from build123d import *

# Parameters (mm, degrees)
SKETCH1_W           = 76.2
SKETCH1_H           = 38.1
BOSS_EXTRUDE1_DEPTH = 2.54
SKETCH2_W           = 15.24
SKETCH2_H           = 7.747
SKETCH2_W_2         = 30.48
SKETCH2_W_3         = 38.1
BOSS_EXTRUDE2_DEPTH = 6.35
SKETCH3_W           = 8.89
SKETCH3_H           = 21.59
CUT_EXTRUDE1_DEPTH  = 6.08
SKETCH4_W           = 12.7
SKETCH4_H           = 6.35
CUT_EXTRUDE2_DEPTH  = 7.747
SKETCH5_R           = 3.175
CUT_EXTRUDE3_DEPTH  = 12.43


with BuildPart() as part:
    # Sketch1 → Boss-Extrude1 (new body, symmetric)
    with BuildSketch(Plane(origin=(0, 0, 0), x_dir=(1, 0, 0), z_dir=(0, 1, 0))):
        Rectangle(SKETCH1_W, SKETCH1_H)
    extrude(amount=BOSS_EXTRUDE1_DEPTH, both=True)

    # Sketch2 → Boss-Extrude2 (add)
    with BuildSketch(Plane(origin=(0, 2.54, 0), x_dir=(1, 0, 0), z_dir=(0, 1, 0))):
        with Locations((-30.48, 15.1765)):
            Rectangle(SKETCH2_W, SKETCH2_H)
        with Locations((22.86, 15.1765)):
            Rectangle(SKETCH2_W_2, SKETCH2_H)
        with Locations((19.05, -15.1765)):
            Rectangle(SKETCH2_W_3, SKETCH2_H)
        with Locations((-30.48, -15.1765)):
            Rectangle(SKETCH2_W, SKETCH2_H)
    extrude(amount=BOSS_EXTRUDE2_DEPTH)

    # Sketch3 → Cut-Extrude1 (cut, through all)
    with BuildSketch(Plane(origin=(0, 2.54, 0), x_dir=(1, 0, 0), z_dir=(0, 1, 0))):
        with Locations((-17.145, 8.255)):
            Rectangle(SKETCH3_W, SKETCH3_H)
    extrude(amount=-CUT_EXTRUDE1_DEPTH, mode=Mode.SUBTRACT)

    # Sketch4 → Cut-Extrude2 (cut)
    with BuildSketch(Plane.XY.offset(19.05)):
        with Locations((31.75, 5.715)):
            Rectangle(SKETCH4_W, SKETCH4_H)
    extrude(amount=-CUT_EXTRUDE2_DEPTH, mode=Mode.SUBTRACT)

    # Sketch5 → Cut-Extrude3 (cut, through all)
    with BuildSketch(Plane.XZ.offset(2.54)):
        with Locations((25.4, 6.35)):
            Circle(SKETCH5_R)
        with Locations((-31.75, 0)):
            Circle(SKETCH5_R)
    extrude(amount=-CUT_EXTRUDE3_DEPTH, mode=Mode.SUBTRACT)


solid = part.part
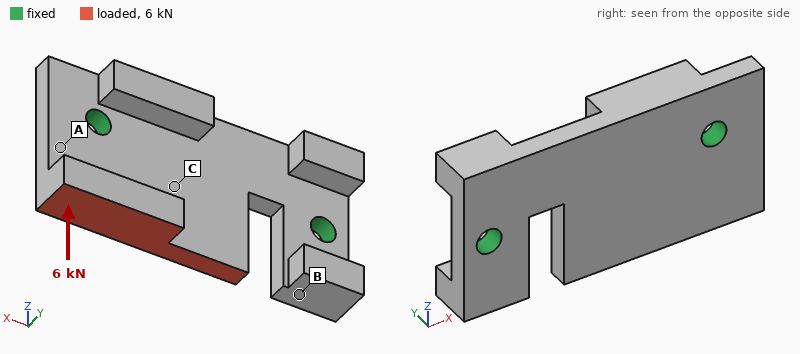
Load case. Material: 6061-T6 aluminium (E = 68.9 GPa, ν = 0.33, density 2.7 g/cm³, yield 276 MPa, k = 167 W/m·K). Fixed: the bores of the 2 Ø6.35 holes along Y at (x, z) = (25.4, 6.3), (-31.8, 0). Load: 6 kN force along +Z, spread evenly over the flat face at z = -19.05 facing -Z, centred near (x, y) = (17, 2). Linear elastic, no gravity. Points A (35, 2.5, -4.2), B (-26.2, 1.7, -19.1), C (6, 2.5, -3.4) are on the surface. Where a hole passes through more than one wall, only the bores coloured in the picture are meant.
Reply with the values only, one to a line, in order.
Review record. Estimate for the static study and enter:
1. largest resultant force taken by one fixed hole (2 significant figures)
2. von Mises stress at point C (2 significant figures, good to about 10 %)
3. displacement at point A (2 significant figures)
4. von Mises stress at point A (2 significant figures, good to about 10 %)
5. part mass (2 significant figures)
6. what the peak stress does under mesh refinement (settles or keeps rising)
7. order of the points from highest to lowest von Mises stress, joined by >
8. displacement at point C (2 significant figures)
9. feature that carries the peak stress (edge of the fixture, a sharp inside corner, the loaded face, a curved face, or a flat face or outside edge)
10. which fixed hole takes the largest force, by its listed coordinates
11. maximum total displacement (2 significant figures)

5.1 kN
59 MPa
0.029 mm
110 MPa
48 g
keeps rising
A > C > B
0.044 mm
edge of the fixture
(25.4, 6.3)
0.18 mm
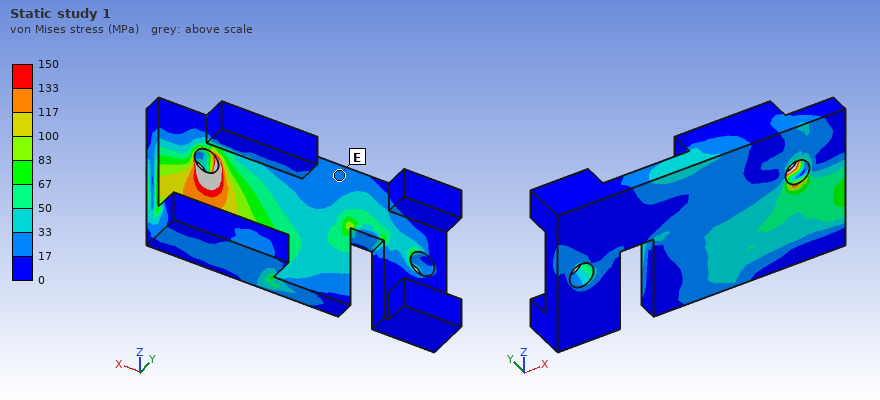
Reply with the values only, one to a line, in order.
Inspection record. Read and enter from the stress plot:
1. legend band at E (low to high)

17 to 33 MPa
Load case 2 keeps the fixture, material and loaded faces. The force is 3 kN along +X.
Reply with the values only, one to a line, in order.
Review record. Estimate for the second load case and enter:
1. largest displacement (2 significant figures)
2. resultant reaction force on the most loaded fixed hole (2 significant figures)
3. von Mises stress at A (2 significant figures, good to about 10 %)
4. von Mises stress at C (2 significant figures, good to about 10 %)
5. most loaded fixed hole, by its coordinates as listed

69 µm
3.5 kN
33 MPa
33 MPa
(25.4, 6.3)
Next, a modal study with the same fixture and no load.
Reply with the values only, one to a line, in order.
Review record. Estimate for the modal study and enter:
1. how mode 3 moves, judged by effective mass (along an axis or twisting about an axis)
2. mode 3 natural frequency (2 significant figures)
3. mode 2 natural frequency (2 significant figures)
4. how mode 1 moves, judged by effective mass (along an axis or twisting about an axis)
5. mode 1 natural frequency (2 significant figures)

along Y
7400 Hz
6000 Hz
along Y
3900 Hz
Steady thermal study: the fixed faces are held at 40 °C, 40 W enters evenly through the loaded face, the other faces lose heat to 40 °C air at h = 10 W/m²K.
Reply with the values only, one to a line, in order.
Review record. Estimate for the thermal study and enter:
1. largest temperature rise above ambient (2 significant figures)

29 K
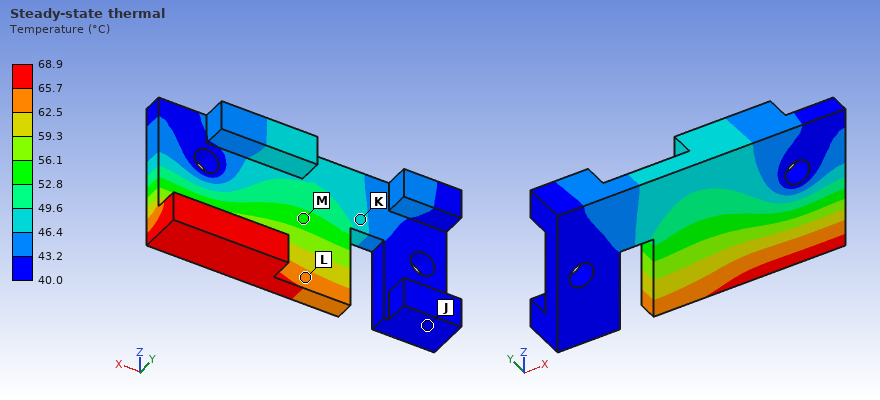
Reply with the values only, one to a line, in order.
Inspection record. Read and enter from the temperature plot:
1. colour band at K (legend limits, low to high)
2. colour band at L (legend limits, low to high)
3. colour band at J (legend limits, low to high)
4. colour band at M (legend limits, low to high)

46.4 to 49.6 °C
62.5 to 65.7 °C
40.0 to 43.2 °C
52.8 to 56.1 °C
